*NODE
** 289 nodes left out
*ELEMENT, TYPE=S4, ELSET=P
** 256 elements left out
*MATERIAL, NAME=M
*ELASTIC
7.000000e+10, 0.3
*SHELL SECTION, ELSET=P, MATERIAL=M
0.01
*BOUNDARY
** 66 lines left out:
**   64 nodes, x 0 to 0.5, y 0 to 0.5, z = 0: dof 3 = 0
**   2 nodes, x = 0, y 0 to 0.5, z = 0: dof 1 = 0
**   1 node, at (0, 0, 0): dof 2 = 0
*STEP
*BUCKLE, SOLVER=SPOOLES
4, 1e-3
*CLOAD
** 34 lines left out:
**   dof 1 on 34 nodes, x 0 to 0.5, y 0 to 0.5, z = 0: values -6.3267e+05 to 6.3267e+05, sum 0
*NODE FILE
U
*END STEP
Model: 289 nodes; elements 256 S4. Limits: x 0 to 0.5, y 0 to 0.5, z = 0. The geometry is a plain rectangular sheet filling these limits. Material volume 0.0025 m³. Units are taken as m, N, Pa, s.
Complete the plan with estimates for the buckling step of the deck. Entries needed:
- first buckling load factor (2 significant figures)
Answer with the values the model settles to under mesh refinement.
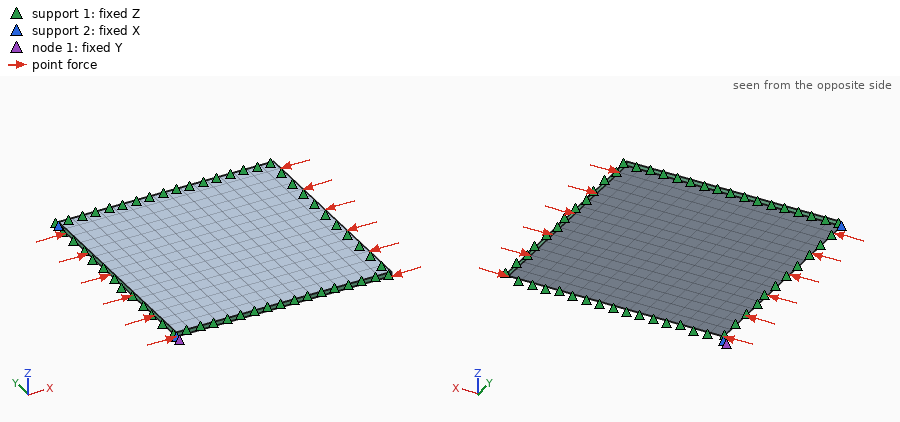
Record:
0.049
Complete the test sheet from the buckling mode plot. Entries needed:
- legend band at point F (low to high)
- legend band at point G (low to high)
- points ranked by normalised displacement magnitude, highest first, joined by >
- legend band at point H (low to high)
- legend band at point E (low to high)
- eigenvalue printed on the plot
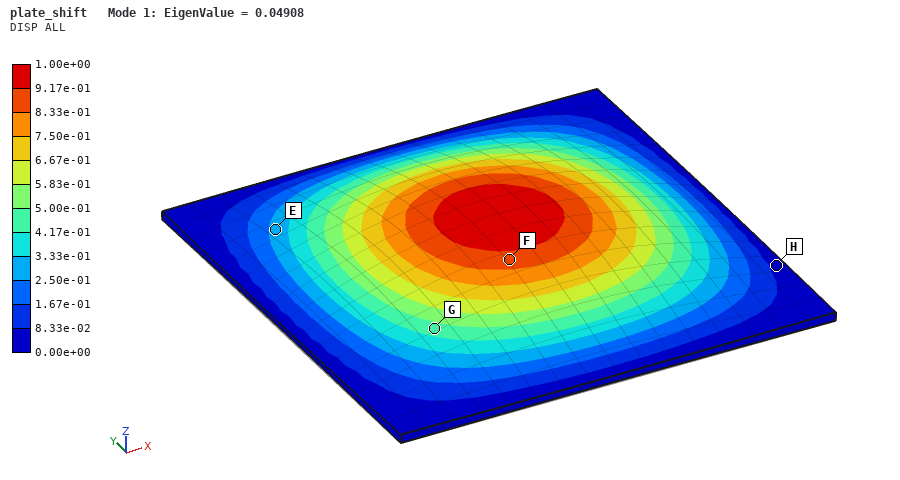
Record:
8.33e-01 to 9.17e-01
4.17e-01 to 5.00e-01
F > G > E > H
0.00e+00 to 8.33e-02
2.50e-01 to 3.33e-01
0.04908
